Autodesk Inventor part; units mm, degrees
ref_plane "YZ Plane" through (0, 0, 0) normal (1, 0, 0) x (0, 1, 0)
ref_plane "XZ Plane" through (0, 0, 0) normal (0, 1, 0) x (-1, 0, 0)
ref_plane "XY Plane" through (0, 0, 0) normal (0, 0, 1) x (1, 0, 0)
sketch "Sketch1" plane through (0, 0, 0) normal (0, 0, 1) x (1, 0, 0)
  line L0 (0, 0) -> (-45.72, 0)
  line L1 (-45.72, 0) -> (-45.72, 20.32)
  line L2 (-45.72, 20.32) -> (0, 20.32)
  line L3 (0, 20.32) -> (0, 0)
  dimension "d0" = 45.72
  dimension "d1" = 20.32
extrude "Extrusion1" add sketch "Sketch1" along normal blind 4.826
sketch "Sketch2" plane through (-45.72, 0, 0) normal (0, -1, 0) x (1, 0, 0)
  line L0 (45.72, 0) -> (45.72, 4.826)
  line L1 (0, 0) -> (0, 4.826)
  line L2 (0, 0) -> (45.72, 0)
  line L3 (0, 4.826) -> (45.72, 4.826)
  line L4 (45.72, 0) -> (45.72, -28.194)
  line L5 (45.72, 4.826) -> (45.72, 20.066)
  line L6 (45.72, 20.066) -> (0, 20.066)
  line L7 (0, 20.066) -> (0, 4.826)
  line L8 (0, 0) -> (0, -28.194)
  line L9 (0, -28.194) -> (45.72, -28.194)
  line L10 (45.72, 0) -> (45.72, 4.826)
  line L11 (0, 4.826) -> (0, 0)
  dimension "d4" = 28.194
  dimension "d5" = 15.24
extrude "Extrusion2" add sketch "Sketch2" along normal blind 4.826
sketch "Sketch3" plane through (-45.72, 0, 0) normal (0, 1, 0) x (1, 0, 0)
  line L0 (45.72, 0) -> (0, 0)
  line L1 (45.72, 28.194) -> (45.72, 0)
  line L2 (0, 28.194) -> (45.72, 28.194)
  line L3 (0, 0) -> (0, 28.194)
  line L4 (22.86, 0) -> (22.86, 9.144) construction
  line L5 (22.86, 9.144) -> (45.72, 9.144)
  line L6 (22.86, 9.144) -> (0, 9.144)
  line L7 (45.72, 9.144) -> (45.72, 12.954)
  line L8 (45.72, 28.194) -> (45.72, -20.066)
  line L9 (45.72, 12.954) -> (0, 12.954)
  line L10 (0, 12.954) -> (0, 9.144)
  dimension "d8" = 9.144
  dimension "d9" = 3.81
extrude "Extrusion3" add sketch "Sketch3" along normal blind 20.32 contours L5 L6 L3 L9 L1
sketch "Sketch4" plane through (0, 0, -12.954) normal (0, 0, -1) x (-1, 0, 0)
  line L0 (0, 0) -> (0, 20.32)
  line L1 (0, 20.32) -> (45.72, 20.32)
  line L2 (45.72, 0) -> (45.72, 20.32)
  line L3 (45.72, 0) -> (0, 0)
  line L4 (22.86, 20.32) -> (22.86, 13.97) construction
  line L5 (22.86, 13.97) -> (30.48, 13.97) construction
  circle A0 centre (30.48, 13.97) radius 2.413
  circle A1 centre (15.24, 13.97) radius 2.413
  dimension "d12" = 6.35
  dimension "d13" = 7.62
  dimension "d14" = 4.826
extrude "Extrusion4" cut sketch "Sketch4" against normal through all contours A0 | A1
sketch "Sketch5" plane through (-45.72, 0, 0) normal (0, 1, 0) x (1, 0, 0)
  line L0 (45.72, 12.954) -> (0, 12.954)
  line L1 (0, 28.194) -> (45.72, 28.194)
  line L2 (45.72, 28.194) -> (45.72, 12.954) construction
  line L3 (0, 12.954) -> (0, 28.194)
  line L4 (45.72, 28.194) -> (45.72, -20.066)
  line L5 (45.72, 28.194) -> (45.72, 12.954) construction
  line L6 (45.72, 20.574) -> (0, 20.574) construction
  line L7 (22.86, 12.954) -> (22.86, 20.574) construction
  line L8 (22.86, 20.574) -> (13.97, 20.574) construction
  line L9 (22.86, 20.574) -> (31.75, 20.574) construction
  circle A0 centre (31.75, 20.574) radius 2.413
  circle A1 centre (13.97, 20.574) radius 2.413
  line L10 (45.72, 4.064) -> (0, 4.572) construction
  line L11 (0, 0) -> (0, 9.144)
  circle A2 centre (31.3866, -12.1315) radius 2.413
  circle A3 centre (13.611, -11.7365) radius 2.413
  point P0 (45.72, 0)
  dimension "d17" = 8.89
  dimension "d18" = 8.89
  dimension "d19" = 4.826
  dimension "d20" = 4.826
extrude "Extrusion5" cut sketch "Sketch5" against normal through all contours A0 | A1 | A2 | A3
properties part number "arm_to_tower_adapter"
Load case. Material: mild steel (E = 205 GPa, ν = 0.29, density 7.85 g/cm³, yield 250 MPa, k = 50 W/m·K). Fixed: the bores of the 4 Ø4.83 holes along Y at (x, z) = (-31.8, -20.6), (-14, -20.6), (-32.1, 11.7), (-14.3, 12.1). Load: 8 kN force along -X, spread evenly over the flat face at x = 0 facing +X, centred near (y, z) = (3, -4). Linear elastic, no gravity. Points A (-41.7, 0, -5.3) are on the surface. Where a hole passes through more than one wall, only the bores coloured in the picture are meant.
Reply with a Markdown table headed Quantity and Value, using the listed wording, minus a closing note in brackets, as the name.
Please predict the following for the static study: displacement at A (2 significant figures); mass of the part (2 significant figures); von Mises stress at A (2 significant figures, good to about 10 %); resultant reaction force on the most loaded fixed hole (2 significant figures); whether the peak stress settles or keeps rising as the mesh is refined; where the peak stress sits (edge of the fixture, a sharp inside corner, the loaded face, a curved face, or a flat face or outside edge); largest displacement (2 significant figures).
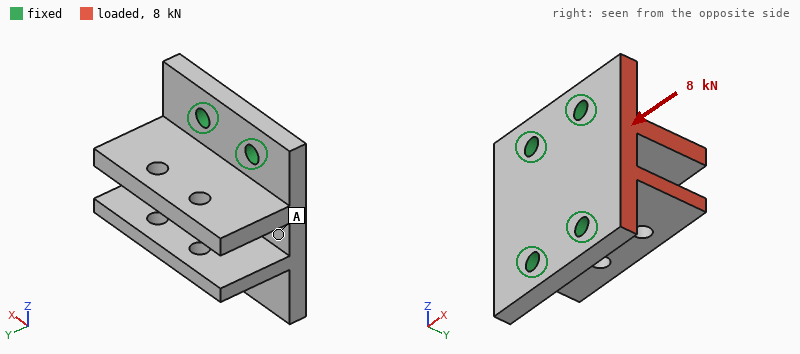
| Quantity | Value |
|---|---|
| displacement at A | 8.4 µm |
| mass of the part | 140 g |
| von Mises stress at A | 15 MPa |
| resultant reaction force on the most loaded fixed hole | 2.9 kN |
| whether the peak stress settles or keeps rising as the mesh is refined | keeps rising |
| where the peak stress sits | edge of the fixture |
| largest displacement | 19 µm |
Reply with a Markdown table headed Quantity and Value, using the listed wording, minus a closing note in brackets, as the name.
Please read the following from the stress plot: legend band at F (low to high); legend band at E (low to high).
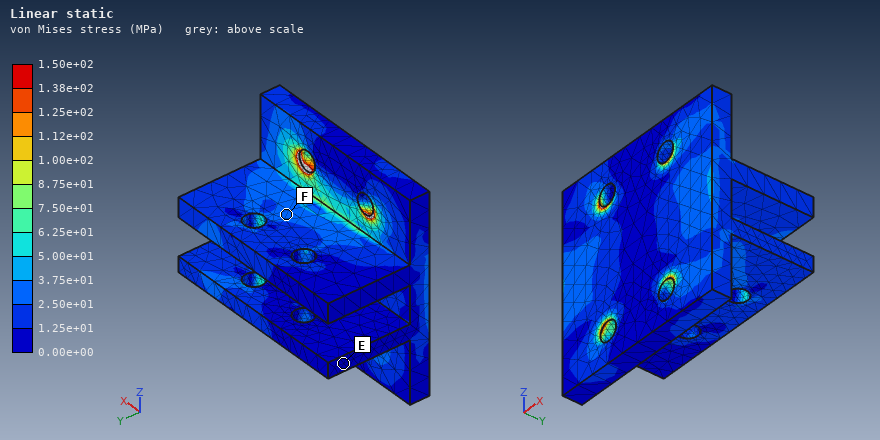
| Quantity | Value |
|---|---|
| legend band at F | 2.50e+01 to 3.75e+01 MPa |
| legend band at E | 0.00e+00 to 1.25e+01 MPa |
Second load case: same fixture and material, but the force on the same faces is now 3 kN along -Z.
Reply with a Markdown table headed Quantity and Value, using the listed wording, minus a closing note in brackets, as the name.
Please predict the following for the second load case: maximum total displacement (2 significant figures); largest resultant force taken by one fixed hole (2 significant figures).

| Quantity | Value |
|---|---|
| maximum total displacement | 54 µm |
| largest resultant force taken by one fixed hole | 1.9 kN |
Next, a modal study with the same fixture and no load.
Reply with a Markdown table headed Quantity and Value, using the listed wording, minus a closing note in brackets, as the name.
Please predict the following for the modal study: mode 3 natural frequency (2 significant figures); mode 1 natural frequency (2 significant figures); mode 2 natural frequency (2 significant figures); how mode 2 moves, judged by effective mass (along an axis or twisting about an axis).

| Quantity | Value |
|---|---|
| mode 3 natural frequency | 8300 Hz |
| mode 1 natural frequency | 6100 Hz |
| mode 2 natural frequency | 7500 Hz |
| how mode 2 moves, judged by effective mass | along Z |
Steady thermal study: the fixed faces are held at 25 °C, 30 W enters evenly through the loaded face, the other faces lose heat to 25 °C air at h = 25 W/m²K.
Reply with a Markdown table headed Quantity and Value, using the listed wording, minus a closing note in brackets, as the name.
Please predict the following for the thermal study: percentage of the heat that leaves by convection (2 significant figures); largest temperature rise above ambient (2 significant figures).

| Quantity | Value |
|---|---|
| percentage of the heat that leaves by convection | 8.5 % |
| largest temperature rise above ambient | 39 K |
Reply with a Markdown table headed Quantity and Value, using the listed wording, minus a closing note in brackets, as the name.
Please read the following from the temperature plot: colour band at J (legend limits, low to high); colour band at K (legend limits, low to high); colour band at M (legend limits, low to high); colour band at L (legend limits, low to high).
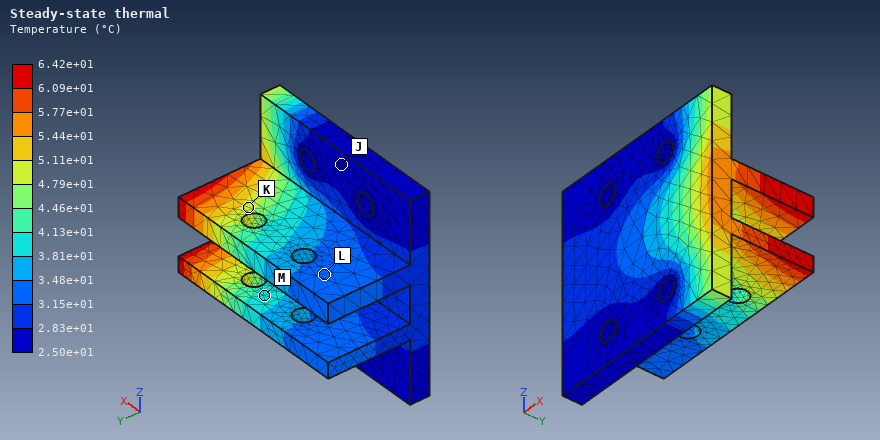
| Quantity | Value |
|---|---|
| colour band at J | 2.50e+01 to 2.83e+01 °C |
| colour band at K | 4.79e+01 to 5.11e+01 °C |
| colour band at M | 3.81e+01 to 4.13e+01 °C |
| colour band at L | 3.15e+01 to 3.48e+01 °C |
